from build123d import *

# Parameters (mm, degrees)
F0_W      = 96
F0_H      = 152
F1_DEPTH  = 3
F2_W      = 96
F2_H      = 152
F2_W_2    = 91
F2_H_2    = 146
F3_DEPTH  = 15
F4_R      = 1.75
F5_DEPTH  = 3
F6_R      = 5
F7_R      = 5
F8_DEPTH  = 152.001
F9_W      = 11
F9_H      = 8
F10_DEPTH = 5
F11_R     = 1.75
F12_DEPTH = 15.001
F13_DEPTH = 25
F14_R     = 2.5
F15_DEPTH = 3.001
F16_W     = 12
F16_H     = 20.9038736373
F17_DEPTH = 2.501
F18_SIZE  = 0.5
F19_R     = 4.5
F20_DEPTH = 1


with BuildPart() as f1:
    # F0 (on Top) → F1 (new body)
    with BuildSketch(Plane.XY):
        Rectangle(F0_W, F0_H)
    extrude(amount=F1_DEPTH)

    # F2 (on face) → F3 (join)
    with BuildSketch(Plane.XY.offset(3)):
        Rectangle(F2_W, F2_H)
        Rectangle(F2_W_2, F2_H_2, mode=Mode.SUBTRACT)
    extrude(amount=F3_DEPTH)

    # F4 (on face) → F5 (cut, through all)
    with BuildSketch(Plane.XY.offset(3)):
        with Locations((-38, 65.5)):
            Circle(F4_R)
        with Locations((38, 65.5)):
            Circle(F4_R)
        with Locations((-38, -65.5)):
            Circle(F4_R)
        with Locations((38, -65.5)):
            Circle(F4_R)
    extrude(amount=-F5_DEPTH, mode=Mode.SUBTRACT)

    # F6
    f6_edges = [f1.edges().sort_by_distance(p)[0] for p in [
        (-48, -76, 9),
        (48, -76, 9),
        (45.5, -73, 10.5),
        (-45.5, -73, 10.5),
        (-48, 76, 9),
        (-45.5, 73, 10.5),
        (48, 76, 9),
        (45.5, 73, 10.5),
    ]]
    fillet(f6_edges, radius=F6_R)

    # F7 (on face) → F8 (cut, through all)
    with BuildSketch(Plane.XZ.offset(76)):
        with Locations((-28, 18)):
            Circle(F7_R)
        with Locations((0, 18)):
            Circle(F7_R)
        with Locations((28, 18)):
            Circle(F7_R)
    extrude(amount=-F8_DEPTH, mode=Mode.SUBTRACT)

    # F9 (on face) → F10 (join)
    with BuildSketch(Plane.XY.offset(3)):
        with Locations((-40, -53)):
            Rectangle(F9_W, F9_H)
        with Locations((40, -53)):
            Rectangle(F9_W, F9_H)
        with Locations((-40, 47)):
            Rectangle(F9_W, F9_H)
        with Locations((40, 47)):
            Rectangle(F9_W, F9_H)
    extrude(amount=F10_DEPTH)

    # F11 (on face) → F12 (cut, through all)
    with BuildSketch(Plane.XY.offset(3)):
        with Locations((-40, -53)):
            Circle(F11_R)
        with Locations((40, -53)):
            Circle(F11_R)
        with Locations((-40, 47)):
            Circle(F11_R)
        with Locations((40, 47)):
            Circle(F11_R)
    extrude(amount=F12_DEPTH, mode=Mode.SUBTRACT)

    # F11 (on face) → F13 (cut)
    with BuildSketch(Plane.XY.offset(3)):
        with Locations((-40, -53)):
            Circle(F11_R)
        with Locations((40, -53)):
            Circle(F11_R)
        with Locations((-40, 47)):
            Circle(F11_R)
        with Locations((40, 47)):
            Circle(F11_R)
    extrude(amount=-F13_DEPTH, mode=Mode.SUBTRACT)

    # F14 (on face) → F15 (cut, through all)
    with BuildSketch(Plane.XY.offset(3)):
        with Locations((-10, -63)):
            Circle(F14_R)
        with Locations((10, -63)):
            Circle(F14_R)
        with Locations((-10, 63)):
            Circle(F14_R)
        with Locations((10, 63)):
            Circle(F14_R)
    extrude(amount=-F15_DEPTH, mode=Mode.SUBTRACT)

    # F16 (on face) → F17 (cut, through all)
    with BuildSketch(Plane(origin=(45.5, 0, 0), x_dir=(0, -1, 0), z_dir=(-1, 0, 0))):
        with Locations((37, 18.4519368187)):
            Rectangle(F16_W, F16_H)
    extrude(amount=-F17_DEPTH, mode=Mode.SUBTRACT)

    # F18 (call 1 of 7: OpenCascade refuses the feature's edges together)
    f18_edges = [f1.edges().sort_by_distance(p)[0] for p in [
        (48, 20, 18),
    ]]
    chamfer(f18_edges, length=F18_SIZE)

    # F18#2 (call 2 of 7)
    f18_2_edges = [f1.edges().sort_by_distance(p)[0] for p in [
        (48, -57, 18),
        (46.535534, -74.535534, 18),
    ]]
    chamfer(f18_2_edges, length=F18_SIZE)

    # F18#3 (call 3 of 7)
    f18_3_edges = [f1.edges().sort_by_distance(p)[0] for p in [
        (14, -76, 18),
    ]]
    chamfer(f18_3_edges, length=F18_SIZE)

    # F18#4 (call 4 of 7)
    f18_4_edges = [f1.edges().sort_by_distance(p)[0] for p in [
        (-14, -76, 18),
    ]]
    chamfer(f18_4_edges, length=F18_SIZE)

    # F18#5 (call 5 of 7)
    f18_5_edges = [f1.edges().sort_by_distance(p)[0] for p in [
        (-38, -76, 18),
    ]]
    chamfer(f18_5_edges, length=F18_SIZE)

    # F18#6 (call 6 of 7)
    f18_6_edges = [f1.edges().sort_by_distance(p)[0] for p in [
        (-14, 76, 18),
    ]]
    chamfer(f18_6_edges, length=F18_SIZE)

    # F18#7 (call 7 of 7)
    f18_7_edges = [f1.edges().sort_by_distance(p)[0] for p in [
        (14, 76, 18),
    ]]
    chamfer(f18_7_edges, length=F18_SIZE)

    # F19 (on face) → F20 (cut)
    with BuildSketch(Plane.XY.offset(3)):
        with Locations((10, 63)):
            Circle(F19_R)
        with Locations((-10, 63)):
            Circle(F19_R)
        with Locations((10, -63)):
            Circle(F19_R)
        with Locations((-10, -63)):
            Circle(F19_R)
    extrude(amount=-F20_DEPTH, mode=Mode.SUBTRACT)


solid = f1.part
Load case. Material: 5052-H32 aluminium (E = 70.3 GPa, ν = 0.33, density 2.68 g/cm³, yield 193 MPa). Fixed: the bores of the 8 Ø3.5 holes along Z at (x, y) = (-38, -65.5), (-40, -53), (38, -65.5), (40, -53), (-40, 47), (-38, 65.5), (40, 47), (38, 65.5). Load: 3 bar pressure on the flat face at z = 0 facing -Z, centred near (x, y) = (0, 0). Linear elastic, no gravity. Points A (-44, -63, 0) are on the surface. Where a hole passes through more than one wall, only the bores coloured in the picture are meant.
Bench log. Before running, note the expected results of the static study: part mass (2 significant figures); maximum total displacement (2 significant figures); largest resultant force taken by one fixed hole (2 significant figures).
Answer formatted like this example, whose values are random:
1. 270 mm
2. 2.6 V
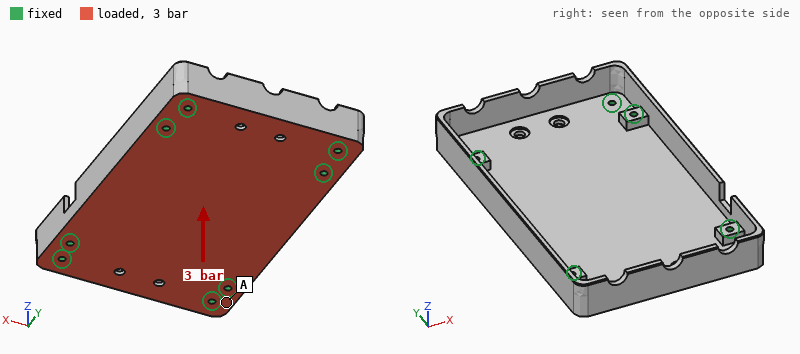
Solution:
1. 170 g
2. 0.50 mm
3. 1.2 kN
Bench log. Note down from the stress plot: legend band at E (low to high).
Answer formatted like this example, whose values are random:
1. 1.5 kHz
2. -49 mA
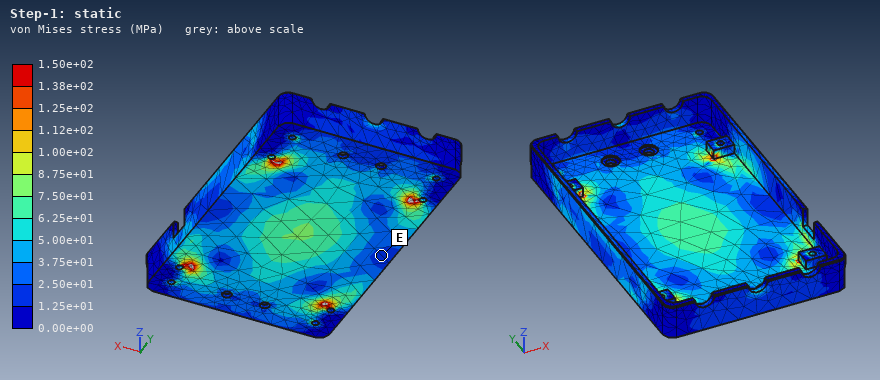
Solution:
1. 1.25e+01 to 2.50e+01 MPa
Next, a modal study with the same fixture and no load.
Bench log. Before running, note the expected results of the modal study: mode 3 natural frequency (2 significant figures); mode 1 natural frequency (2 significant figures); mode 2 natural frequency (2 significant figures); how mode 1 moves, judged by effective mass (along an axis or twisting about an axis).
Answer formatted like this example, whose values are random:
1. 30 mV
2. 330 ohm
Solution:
1. 3800 Hz
2. 1700 Hz
3. 3200 Hz
4. along Z
